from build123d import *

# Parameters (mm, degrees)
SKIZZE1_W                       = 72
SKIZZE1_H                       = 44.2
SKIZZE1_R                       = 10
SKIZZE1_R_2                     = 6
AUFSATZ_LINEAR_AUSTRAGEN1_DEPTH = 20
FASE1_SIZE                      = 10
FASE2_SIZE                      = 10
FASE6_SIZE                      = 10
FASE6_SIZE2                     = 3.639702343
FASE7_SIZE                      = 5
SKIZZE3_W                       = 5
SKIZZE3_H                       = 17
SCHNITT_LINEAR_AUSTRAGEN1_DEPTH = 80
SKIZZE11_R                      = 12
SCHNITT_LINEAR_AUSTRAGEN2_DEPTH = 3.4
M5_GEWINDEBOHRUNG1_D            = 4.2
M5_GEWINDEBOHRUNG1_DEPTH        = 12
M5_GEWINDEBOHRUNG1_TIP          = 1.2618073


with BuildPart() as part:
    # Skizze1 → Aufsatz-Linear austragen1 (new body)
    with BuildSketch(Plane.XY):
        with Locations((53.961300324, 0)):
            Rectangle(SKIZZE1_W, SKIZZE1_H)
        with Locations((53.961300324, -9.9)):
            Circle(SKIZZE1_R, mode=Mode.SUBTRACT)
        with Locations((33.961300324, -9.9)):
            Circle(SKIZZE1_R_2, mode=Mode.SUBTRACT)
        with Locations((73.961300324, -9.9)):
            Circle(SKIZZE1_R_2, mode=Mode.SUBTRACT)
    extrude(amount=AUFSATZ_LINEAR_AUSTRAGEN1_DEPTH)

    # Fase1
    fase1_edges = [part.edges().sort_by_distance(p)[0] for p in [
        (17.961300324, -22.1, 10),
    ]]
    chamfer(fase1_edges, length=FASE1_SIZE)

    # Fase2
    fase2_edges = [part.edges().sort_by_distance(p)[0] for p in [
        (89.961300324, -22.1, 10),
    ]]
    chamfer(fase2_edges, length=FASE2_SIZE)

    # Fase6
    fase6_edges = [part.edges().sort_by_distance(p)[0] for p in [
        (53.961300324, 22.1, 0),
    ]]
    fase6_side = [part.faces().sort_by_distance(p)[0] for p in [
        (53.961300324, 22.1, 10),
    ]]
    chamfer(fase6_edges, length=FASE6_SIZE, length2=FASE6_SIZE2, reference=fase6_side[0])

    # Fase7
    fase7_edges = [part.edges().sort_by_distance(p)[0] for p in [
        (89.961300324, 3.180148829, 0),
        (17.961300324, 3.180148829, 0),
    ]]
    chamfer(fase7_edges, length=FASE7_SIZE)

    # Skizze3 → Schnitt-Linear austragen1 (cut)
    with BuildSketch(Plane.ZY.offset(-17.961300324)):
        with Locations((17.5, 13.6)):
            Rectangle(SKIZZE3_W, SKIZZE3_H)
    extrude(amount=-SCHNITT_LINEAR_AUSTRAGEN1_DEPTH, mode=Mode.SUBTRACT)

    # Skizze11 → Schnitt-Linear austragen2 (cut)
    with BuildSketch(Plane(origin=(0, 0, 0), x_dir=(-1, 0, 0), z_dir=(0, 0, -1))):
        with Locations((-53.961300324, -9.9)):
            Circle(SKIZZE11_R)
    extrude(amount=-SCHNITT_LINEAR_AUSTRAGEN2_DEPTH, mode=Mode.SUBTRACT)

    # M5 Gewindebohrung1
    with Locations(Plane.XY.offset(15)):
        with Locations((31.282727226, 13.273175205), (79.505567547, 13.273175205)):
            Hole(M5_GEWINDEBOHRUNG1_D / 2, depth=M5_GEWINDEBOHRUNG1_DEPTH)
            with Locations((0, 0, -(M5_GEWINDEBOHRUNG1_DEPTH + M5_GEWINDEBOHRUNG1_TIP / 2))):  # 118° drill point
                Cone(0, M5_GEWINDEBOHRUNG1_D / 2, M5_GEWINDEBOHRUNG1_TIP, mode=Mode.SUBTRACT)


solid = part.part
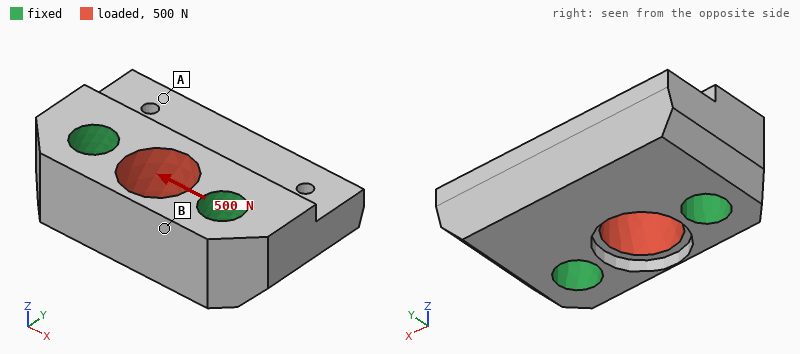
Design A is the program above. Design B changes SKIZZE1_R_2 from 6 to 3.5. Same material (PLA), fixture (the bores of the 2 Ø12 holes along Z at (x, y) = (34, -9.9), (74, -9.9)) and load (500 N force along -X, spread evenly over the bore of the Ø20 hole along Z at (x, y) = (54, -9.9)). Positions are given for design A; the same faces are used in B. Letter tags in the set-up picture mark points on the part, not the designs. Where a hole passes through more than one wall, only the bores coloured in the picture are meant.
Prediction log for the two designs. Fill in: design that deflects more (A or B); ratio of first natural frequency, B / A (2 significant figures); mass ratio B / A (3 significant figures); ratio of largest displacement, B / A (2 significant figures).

B
0.83
1.07
1.2
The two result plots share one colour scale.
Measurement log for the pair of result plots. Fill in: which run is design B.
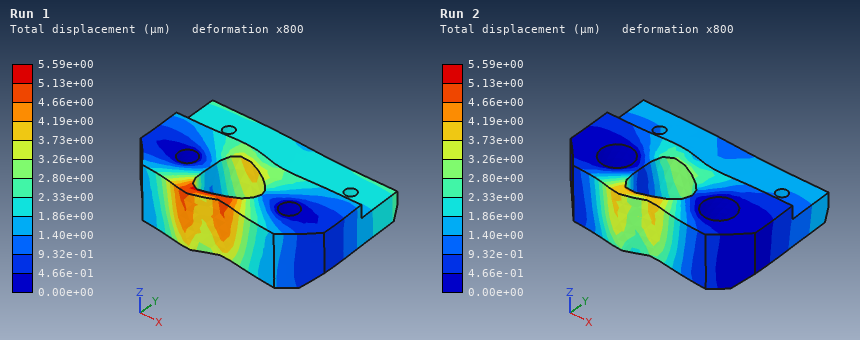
Run 1
